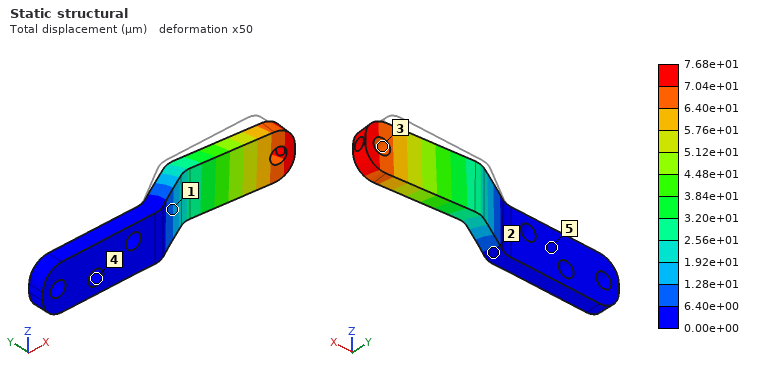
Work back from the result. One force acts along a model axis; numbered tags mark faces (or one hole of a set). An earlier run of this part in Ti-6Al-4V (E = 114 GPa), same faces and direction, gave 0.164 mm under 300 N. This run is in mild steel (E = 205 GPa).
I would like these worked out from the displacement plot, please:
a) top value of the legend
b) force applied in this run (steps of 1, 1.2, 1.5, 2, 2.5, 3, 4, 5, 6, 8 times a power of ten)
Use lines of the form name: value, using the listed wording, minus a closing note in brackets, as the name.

top value of the legend: 7.68e+01 µm
force applied in this run: 250 N
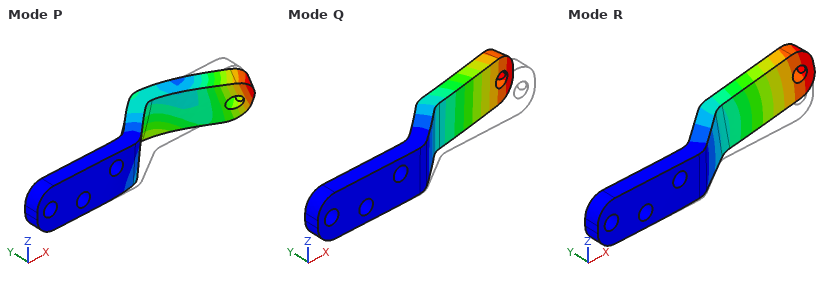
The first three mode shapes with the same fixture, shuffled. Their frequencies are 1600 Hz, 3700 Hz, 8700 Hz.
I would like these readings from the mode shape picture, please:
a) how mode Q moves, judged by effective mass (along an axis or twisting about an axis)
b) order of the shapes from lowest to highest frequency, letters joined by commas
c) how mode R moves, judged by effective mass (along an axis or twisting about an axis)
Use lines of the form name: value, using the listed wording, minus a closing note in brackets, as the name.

how mode Q moves, judged by effective mass: along Y
order of the shapes from lowest to highest frequency, letters joined by commas: Q, R, P
how mode R moves, judged by effective mass: along Z
